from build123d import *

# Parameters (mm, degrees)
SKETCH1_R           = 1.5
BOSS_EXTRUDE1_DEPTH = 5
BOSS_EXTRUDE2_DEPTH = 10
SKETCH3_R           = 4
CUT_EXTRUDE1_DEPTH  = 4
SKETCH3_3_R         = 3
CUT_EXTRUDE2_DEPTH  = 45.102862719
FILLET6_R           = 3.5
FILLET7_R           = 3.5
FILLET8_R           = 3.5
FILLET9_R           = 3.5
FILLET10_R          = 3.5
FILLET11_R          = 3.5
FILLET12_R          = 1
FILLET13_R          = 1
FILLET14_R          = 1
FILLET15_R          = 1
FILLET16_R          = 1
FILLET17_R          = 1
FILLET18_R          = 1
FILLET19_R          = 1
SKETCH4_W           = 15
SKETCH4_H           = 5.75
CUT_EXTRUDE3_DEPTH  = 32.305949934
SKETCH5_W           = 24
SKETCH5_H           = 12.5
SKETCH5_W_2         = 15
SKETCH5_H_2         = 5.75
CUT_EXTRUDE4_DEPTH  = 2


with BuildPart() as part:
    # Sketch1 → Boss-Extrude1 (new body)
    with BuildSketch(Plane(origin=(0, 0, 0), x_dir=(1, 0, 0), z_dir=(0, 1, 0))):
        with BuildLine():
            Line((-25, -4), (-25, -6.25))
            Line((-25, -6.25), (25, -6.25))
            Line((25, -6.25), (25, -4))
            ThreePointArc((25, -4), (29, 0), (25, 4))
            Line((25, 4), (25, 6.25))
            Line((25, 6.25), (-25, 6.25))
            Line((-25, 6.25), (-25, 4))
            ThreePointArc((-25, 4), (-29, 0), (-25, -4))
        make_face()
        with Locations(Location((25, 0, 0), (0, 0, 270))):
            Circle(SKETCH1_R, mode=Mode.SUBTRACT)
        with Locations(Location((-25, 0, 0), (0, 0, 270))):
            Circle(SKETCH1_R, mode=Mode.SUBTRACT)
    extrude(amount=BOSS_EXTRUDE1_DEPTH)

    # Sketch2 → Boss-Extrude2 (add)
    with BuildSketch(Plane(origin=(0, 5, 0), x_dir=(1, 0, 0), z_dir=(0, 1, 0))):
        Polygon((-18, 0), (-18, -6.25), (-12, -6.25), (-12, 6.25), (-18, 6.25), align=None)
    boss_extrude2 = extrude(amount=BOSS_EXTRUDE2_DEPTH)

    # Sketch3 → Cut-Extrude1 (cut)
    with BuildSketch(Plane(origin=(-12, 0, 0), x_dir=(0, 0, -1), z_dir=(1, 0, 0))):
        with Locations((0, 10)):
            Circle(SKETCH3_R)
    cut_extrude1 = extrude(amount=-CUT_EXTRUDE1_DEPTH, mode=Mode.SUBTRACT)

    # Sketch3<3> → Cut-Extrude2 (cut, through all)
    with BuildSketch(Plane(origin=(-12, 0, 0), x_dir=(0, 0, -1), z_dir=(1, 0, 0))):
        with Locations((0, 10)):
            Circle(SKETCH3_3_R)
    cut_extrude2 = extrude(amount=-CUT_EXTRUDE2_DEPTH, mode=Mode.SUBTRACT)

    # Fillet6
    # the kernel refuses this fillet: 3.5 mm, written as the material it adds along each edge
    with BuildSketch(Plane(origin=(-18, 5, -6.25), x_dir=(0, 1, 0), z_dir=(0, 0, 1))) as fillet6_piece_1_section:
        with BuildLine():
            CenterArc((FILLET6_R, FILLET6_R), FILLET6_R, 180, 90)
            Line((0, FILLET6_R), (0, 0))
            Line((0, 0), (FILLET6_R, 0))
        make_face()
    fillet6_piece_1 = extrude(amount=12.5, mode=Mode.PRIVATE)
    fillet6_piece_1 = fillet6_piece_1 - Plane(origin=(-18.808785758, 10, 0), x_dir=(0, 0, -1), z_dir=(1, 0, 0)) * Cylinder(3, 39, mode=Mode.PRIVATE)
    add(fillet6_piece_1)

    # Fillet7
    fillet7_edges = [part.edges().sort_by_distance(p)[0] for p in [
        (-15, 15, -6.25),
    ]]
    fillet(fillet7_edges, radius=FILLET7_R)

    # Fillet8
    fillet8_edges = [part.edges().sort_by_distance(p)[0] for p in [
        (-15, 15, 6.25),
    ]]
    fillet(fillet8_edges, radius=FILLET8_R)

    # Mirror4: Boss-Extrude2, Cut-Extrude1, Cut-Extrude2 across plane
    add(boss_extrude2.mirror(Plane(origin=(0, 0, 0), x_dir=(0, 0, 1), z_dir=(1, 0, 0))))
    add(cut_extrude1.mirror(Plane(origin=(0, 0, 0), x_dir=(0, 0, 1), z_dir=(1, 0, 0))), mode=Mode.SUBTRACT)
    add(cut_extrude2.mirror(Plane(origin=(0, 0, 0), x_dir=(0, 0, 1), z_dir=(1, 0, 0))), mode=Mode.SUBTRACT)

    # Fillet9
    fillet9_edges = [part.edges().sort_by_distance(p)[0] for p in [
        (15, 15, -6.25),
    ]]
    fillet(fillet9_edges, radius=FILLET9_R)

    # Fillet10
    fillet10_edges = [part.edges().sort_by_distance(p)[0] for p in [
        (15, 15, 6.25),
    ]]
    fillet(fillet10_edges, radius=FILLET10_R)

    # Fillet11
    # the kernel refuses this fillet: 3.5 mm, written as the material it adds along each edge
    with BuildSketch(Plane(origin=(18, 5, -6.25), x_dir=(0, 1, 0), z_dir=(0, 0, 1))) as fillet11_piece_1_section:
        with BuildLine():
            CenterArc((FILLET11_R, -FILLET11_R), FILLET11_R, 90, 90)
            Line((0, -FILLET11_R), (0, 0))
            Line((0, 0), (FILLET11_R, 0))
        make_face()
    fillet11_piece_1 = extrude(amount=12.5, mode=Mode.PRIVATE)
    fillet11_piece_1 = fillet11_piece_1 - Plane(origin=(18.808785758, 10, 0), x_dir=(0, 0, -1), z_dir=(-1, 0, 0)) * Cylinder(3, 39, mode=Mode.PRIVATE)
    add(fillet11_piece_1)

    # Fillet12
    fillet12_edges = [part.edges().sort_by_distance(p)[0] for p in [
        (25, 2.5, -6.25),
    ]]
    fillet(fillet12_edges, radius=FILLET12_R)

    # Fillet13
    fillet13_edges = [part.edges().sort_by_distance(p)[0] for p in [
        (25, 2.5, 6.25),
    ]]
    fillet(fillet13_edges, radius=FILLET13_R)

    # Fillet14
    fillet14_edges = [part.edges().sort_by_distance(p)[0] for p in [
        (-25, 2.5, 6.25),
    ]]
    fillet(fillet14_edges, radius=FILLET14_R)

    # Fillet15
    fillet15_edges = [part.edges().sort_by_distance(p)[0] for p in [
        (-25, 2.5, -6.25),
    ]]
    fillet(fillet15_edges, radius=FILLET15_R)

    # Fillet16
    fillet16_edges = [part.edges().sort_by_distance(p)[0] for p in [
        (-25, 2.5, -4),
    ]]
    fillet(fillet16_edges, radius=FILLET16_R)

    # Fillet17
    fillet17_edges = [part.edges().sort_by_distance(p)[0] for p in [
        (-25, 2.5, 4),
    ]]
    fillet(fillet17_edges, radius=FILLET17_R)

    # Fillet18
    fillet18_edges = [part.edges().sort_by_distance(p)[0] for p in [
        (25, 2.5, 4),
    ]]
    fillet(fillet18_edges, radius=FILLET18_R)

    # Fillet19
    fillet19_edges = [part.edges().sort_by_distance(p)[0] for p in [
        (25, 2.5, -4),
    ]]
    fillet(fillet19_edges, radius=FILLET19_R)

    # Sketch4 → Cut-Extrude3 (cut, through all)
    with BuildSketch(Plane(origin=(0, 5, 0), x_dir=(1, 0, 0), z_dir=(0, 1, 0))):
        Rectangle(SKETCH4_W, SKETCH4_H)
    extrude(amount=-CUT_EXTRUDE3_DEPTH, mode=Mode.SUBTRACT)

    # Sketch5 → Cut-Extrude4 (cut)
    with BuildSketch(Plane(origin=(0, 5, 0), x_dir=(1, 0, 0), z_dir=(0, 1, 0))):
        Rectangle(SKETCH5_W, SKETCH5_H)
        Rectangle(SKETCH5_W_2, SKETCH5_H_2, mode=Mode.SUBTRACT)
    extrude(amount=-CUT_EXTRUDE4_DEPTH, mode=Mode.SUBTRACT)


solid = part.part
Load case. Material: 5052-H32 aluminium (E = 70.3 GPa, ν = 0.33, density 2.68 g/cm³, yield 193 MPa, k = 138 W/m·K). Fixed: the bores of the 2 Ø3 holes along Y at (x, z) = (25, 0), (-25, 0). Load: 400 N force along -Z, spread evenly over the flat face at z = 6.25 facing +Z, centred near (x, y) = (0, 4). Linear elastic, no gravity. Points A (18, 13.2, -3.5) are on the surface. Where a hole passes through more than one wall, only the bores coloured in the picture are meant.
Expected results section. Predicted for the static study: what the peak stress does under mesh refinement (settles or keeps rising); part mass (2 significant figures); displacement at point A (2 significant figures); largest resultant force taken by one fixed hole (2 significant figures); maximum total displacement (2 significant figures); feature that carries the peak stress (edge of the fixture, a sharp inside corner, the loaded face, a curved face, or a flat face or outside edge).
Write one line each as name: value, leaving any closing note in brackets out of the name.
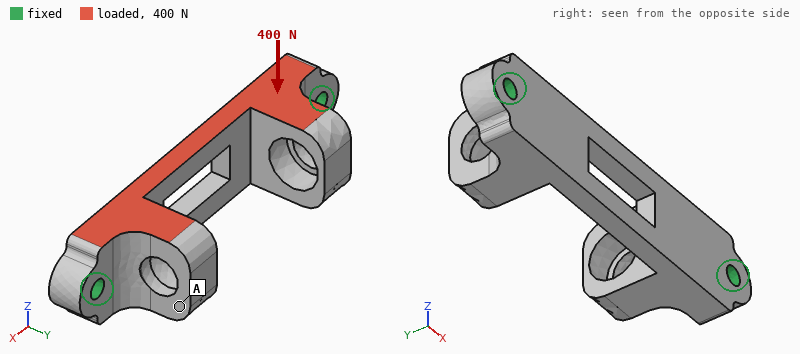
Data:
what the peak stress does under mesh refinement: keeps rising
part mass: 9.2 g
displacement at point A: 5.4 µm
largest resultant force taken by one fixed hole: 200 N
maximum total displacement: 10 µm
feature that carries the peak stress: edge of the fixture
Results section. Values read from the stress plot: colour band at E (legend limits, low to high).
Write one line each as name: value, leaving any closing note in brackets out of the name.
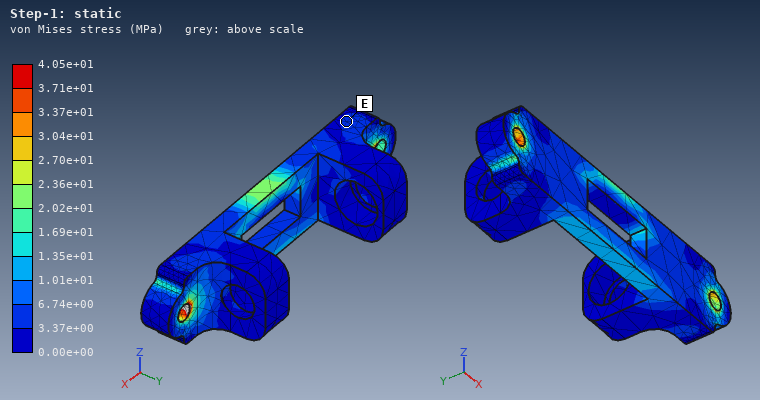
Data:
colour band at E: 3.37e+00 to 6.74e+00 MPa
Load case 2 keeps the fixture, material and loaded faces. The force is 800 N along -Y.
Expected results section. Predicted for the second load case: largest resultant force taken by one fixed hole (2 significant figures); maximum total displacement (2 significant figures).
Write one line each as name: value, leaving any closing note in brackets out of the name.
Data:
largest resultant force taken by one fixed hole: 450 N
maximum total displacement: 70 µm
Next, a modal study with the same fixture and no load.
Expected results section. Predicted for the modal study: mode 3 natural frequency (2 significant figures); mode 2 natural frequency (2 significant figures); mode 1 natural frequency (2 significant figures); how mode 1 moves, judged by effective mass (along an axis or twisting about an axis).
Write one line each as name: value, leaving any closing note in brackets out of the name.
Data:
mode 3 natural frequency: 14 kHz
mode 2 natural frequency: 13 kHz
mode 1 natural frequency: 9300 Hz
how mode 1 moves, judged by effective mass: along Y
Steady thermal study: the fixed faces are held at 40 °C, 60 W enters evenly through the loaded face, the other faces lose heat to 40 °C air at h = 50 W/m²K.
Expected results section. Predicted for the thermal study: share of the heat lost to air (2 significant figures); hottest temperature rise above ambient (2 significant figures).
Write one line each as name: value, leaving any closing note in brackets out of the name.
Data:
share of the heat lost to air: 5.1 %
hottest temperature rise above ambient: 61 K
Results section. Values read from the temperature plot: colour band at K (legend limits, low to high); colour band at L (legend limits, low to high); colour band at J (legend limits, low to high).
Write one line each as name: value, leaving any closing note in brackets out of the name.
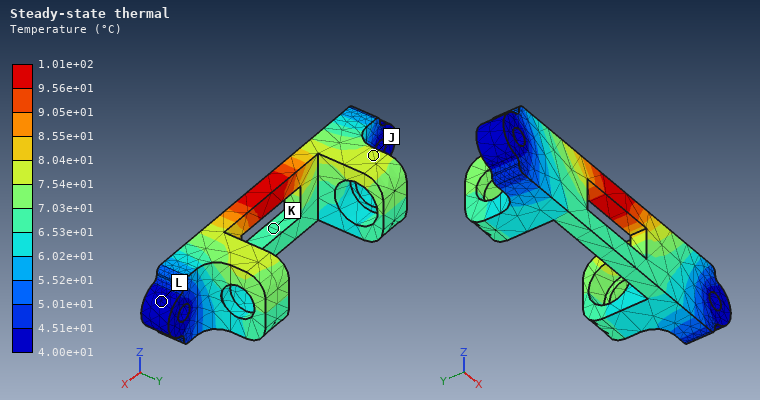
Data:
colour band at K: 6.53e+01 to 7.03e+01 °C
colour band at L: 4.00e+01 to 4.51e+01 °C
colour band at J: 7.54e+01 to 8.04e+01 °C
